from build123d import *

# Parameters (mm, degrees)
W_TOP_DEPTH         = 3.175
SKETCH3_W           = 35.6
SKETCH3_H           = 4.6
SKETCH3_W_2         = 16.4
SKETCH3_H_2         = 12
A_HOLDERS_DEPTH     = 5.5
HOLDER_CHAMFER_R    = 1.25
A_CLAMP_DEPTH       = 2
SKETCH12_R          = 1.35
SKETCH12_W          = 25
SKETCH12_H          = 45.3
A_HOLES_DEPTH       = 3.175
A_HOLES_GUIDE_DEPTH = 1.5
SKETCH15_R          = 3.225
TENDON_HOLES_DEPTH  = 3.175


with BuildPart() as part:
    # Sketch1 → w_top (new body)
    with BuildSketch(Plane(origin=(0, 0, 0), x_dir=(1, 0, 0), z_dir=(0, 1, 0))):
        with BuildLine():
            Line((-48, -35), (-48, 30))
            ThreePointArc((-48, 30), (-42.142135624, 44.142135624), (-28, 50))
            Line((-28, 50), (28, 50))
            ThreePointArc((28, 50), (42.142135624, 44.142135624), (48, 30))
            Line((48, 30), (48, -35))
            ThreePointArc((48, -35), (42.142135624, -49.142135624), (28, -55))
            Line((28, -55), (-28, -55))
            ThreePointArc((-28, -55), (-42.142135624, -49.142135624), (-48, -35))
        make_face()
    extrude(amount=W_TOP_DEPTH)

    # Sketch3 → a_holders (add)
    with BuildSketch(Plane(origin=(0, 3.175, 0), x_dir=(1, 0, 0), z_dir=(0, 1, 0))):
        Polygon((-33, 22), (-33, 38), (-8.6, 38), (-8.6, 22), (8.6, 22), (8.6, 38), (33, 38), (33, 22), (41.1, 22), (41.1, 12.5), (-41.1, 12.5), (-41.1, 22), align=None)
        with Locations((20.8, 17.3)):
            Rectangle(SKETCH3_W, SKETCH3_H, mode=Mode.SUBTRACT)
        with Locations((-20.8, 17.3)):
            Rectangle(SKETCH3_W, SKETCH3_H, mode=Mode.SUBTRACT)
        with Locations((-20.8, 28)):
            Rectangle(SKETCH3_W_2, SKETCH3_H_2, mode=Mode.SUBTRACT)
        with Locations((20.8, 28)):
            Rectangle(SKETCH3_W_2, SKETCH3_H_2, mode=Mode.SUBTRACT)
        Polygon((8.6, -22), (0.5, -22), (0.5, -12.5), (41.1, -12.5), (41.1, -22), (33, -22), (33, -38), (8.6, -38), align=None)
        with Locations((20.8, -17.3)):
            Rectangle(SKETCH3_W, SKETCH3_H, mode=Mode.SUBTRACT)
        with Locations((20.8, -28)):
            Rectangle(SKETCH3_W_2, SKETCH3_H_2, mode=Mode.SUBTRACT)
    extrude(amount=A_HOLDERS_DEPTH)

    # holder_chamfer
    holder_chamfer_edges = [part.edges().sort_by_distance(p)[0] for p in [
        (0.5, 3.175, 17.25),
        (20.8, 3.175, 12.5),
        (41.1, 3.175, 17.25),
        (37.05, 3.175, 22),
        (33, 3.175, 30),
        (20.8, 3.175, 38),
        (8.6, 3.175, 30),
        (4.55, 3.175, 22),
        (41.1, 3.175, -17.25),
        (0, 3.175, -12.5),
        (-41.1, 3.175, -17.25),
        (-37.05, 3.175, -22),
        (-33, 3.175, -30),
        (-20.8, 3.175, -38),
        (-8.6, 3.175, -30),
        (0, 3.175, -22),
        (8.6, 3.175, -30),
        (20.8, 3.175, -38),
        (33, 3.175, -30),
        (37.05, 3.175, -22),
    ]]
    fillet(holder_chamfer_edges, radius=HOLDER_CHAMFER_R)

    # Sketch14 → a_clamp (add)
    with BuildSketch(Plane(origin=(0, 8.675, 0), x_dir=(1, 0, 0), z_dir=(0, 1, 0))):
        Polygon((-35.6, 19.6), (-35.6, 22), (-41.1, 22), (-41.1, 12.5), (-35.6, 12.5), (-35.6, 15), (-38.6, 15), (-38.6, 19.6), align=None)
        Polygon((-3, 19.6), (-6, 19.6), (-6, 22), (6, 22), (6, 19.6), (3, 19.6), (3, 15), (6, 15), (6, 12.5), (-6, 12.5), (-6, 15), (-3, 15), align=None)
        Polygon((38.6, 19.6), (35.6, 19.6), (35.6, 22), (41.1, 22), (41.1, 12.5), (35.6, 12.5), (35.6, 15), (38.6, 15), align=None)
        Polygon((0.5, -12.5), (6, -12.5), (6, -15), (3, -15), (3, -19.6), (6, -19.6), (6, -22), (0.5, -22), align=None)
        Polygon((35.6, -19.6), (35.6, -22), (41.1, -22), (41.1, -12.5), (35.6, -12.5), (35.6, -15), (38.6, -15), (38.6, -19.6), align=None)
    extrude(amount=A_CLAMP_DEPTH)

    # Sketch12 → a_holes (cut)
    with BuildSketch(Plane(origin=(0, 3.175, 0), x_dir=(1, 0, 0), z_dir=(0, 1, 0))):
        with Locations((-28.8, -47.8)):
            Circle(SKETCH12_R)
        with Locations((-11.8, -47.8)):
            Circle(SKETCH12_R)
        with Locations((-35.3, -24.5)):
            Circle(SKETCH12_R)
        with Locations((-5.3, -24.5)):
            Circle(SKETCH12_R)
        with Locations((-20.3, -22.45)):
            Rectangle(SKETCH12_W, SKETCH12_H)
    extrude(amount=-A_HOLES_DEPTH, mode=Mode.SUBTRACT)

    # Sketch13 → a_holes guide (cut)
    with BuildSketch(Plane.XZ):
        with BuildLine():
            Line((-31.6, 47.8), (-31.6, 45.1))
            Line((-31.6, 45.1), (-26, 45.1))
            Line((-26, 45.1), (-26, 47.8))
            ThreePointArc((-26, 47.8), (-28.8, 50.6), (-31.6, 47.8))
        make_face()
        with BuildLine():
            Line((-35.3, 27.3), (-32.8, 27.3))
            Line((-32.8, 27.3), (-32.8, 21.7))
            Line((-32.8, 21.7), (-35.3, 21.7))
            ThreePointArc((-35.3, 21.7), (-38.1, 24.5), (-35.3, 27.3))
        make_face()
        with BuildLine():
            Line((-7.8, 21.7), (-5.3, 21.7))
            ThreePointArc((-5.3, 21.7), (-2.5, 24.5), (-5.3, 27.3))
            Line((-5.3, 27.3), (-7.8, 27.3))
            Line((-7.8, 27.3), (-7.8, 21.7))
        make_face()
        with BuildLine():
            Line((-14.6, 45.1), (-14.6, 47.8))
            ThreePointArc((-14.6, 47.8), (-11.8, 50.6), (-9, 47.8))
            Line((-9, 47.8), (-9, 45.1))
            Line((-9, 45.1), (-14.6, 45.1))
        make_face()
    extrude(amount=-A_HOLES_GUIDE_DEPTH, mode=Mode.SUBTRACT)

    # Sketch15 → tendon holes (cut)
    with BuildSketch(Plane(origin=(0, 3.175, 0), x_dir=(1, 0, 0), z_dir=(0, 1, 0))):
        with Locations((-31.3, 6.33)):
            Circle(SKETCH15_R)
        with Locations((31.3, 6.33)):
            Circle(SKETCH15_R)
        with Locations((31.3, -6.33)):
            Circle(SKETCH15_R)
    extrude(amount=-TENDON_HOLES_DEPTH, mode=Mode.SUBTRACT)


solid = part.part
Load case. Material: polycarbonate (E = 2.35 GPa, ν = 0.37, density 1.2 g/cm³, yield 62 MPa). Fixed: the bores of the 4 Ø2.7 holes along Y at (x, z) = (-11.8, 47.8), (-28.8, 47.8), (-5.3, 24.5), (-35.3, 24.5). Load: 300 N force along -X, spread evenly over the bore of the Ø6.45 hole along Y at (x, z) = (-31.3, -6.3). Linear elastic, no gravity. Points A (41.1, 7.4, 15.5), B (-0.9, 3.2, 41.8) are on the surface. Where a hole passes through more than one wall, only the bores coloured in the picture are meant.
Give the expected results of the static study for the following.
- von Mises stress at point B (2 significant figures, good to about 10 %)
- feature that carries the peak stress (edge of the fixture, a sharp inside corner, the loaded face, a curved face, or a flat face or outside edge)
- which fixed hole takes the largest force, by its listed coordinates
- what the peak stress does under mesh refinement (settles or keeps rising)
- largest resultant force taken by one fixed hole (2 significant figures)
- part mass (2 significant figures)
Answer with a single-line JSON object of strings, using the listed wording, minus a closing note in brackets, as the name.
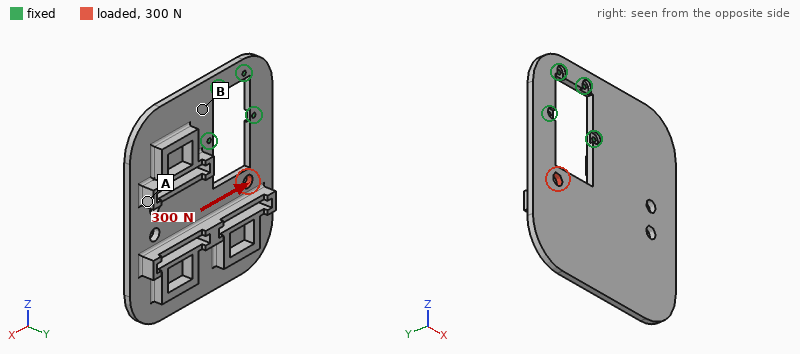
{"von Mises stress at point B": "3.9 MPa", "feature that carries the peak stress": "edge of the fixture", "which fixed hole takes the largest force, by its listed coordinates": "(-5.3, 24.5)", "what the peak stress does under mesh refinement": "keeps rising", "largest resultant force taken by one fixed hole": "380 N", "part mass": "41 g"}
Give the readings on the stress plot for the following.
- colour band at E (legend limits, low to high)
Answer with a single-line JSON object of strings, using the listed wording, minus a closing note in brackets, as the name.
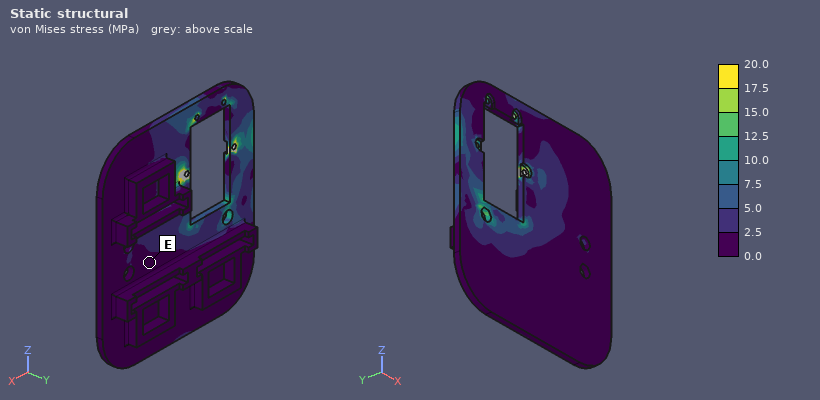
{"colour band at E": "0.0 to 2.5 MPa"}
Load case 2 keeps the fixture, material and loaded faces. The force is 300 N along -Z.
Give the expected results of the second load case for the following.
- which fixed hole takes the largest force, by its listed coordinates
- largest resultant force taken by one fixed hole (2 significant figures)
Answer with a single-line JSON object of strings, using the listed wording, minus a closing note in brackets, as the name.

{"which fixed hole takes the largest force, by its listed coordinates": "(-35.3, 24.5)", "largest resultant force taken by one fixed hole": "190 N"}
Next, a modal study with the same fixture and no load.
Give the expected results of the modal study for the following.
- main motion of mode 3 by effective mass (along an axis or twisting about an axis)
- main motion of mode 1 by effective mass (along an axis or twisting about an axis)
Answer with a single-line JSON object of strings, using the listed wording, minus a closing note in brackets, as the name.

{"main motion of mode 3 by effective mass": "along Y", "main motion of mode 1 by effective mass": "along Y"}
